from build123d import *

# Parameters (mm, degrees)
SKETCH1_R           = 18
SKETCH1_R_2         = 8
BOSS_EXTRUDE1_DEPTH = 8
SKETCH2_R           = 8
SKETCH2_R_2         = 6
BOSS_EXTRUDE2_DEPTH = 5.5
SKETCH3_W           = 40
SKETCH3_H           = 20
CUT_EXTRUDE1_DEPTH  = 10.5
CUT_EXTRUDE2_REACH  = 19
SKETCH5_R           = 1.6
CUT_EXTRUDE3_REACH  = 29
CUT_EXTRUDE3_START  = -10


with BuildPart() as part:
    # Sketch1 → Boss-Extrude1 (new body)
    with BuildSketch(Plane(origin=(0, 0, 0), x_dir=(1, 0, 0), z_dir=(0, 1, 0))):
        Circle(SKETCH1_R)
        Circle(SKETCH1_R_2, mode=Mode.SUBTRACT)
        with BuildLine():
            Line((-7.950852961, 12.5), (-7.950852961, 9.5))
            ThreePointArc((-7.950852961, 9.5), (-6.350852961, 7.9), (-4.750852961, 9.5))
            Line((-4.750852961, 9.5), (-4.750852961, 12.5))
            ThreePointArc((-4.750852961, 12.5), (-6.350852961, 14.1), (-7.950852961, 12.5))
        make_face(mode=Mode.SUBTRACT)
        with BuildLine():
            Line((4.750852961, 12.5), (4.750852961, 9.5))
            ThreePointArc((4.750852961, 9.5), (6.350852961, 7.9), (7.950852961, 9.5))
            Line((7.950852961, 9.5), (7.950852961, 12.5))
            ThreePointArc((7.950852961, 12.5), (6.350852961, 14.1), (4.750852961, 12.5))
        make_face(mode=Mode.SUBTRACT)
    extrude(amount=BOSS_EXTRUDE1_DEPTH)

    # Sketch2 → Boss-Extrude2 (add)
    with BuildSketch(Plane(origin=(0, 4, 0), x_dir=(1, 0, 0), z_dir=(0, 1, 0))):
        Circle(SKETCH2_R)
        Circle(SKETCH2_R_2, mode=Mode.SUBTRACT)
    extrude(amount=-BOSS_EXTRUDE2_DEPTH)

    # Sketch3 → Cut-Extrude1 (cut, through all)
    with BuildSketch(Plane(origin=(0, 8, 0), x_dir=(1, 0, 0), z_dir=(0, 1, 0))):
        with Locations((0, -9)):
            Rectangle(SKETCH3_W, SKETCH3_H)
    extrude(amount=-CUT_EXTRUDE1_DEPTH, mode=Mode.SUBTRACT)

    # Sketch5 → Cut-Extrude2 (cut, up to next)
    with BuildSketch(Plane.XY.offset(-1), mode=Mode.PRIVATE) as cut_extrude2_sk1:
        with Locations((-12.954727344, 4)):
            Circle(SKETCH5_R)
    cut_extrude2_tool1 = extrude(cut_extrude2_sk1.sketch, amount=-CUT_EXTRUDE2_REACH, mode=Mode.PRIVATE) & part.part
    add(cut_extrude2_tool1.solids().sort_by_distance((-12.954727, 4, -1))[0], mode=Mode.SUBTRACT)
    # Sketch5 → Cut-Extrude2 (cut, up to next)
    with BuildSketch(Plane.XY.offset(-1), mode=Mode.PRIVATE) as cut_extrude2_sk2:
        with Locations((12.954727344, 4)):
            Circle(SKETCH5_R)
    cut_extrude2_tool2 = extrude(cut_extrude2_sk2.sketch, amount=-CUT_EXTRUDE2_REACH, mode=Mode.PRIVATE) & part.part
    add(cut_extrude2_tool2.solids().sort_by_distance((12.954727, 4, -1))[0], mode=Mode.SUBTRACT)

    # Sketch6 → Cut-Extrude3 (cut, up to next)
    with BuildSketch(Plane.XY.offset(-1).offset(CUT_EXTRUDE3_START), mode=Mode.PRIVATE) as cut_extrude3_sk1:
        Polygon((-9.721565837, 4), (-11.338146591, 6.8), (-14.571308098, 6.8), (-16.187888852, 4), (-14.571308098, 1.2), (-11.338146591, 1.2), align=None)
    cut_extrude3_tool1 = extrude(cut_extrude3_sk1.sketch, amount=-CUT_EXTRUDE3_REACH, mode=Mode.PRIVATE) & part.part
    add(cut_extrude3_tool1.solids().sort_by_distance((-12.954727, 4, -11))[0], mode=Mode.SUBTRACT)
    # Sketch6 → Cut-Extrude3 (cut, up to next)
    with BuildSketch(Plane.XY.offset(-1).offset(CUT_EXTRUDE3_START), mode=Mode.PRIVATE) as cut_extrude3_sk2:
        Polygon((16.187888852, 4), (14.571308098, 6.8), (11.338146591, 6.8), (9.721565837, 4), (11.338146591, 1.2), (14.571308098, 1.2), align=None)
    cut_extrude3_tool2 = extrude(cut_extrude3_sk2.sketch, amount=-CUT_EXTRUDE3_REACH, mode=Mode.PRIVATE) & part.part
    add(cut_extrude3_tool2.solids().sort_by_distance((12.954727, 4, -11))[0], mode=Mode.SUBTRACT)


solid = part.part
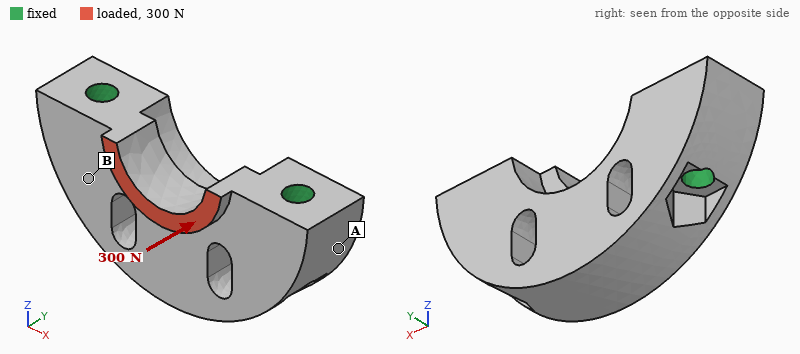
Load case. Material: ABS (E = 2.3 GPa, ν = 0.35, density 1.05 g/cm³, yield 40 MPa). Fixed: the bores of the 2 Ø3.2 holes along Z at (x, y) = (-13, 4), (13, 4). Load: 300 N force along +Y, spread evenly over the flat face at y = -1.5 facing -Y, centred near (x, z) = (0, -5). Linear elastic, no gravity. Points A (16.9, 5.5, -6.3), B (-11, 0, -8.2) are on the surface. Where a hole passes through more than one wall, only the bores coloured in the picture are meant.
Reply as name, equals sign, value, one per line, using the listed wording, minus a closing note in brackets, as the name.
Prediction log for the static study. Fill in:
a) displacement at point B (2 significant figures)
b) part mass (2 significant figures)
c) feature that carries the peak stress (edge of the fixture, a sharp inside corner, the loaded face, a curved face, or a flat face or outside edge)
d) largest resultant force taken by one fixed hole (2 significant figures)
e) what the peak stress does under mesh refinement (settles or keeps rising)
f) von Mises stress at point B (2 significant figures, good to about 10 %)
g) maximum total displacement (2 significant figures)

displacement at point B = 13 µm
part mass = 2.9 g
feature that carries the peak stress = edge of the fixture
largest resultant force taken by one fixed hole = 160 N
what the peak stress does under mesh refinement = keeps rising
von Mises stress at point B = 4.0 MPa
maximum total displacement = 76 µm
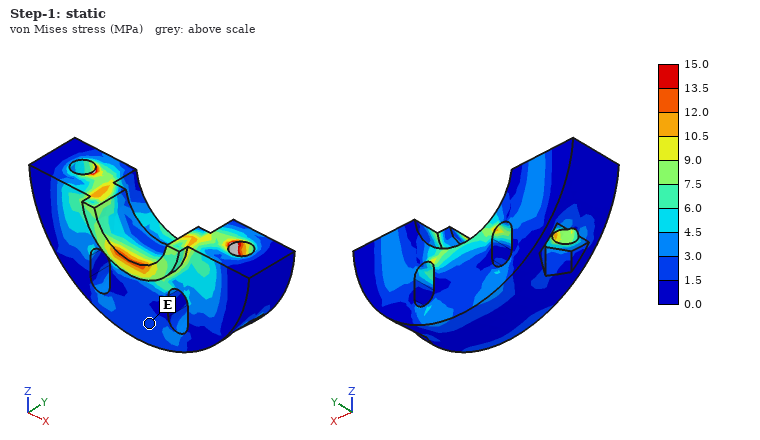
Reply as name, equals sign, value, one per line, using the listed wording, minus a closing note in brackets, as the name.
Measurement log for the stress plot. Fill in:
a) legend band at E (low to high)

legend band at E = 1.5 to 3.0 MPa
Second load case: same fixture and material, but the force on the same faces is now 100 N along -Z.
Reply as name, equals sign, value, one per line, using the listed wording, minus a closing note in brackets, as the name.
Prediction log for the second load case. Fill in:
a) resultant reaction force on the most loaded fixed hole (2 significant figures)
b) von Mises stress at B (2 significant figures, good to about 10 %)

resultant reaction force on the most loaded fixed hole = 55 N
von Mises stress at B = 2.6 MPa
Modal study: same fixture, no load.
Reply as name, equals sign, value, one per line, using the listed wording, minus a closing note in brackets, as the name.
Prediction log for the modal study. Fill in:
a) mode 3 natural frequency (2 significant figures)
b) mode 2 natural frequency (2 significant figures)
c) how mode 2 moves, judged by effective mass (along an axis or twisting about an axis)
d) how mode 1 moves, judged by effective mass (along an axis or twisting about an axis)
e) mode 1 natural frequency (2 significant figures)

mode 3 natural frequency = 15 kHz
mode 2 natural frequency = 13 kHz
how mode 2 moves, judged by effective mass = along Z
how mode 1 moves, judged by effective mass = along Y
mode 1 natural frequency = 7300 Hz
